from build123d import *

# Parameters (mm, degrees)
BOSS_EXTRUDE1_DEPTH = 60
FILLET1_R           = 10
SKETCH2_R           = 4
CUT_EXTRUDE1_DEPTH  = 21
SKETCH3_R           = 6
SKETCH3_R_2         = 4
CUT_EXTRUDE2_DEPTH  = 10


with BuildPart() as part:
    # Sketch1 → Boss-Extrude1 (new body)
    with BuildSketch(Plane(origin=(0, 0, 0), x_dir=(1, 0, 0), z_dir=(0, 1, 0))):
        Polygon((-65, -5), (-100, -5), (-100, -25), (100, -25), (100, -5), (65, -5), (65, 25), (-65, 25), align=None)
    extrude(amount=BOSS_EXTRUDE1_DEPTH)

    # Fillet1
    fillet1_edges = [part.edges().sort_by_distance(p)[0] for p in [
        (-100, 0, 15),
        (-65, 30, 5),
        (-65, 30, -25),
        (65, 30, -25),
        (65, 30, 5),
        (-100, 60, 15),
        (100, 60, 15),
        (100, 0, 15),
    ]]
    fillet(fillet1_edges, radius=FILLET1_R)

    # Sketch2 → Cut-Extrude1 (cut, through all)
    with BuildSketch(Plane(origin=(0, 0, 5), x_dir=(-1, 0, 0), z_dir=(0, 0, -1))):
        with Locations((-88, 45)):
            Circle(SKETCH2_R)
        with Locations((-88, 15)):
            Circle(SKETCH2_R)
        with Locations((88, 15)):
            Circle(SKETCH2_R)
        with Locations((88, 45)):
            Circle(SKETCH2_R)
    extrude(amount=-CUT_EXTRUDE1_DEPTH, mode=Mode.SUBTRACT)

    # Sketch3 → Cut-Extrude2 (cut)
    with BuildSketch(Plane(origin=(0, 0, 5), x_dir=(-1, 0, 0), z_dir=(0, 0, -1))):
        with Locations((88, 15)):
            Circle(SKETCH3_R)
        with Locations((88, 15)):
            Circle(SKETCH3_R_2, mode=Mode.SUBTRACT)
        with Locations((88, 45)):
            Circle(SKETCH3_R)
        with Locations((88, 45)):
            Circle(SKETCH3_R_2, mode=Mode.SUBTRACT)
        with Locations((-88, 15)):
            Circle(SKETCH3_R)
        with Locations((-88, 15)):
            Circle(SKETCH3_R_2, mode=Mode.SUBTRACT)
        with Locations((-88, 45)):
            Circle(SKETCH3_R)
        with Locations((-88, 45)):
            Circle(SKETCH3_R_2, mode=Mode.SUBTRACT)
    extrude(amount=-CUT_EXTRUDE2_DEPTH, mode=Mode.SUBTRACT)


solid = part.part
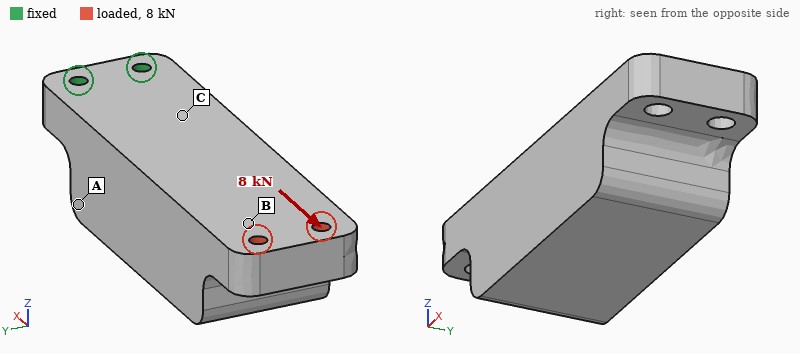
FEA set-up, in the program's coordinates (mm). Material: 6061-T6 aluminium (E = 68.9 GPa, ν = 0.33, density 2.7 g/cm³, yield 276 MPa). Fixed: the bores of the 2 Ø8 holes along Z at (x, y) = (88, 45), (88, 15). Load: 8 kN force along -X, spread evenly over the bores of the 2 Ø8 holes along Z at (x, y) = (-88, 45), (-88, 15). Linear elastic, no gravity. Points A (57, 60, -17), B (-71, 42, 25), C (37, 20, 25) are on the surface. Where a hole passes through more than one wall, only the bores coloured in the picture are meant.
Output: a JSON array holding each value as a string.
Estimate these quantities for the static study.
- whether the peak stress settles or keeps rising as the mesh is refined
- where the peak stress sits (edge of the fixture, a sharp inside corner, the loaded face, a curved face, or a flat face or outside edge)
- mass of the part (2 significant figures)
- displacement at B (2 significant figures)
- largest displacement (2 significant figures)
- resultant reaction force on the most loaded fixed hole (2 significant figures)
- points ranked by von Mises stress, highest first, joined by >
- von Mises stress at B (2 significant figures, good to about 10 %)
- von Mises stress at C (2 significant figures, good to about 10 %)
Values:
["keeps rising", "edge of the fixture", "1.3 kg", "0.089 mm", "0.12 mm", "4.0 kN", "B > C > A", "17 MPa", "10.0 MPa"]
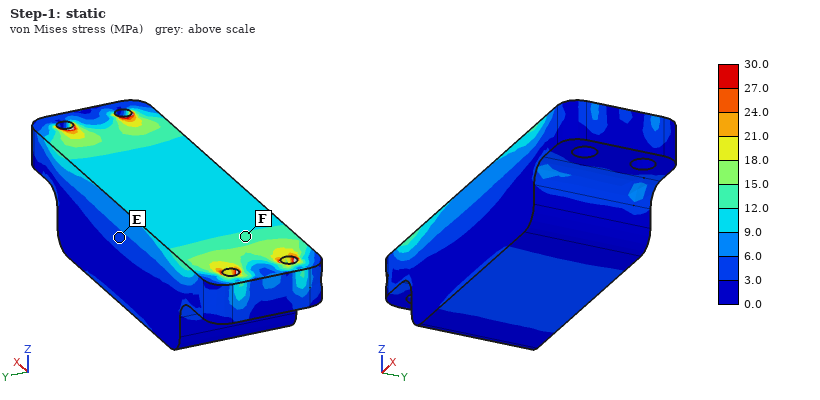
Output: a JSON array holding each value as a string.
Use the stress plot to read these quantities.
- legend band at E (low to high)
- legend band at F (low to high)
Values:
["3.0 to 6.0 MPa", "12.0 to 15.0 MPa"]
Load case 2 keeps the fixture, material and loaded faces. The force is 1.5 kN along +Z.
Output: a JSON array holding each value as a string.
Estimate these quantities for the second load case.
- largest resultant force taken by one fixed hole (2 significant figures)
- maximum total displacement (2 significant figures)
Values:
["990 N", "0.93 mm"]
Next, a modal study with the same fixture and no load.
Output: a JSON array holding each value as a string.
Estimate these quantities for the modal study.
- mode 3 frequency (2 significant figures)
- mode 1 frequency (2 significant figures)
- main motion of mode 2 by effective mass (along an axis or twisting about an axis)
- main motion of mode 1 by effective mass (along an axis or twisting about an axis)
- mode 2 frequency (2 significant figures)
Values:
["2200 Hz", "330 Hz", "along Y", "along Z", "900 Hz"]
